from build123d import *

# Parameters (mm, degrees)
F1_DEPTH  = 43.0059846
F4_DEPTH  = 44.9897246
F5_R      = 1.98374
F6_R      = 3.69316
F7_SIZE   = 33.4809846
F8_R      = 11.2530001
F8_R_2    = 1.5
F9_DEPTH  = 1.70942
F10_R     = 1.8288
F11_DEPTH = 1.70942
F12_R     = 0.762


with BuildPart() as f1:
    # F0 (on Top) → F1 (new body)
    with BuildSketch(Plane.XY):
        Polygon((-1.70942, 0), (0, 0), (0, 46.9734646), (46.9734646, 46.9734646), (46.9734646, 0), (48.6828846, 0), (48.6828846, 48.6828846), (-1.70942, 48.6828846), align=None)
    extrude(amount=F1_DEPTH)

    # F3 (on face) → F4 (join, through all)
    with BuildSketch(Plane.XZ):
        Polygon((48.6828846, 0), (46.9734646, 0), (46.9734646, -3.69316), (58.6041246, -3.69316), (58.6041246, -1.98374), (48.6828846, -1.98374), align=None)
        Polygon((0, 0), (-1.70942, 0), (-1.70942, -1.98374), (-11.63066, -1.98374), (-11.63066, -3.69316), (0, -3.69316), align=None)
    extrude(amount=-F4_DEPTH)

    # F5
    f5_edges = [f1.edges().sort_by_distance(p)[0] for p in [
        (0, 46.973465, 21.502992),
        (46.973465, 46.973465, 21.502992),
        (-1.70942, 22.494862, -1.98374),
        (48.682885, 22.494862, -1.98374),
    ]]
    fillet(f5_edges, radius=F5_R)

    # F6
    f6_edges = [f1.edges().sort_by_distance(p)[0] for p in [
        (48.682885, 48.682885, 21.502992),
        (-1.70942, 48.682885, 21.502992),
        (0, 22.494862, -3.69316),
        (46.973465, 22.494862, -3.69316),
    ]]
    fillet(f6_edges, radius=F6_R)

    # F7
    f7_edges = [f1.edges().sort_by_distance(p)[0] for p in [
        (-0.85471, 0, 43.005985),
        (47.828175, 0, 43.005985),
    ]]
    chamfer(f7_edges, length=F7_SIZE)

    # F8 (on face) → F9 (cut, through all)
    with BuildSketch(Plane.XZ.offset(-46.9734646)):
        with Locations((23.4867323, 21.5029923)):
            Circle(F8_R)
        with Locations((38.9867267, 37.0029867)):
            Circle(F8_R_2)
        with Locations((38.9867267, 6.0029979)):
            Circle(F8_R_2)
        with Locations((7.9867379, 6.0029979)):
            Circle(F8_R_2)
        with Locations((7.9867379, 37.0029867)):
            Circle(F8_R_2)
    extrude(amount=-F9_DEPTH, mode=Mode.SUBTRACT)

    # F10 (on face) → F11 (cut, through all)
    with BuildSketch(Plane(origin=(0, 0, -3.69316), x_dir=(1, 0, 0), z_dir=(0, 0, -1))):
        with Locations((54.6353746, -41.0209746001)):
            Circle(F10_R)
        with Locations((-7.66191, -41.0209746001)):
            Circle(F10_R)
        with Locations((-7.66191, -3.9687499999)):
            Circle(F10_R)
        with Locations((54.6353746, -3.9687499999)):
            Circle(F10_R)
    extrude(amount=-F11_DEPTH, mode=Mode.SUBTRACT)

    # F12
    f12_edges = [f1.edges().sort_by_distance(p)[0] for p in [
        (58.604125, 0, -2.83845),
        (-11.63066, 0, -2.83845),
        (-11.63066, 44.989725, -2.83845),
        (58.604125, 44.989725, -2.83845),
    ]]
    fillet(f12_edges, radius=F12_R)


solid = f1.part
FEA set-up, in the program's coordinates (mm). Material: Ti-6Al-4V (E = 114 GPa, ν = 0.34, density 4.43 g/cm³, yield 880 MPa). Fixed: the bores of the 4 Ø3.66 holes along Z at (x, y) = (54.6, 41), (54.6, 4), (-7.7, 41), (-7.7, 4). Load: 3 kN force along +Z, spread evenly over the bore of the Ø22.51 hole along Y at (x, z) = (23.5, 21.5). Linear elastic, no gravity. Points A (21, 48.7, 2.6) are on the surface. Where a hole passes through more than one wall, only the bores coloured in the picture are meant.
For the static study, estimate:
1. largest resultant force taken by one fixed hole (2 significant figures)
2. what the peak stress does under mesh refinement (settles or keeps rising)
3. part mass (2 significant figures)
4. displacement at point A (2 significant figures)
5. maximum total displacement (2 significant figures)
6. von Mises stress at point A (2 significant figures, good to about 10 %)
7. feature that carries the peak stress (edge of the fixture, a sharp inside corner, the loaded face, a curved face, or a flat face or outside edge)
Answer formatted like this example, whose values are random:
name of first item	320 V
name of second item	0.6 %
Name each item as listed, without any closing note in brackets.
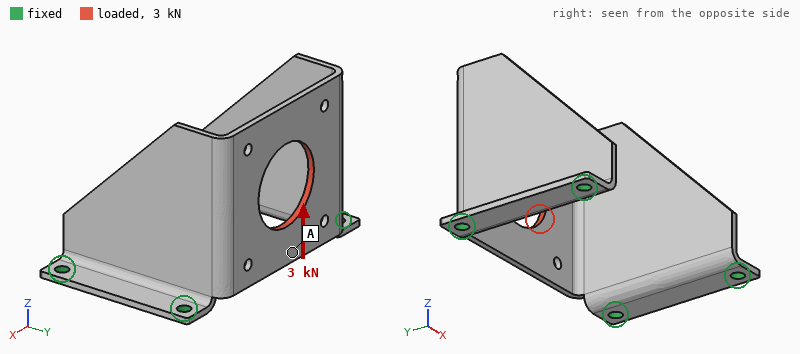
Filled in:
largest resultant force taken by one fixed hole	1.9 kN
what the peak stress does under mesh refinement	keeps rising
part mass	43 g
displacement at point A	0.22 mm
maximum total displacement	0.29 mm
von Mises stress at point A	88 MPa
feature that carries the peak stress	edge of the fixture
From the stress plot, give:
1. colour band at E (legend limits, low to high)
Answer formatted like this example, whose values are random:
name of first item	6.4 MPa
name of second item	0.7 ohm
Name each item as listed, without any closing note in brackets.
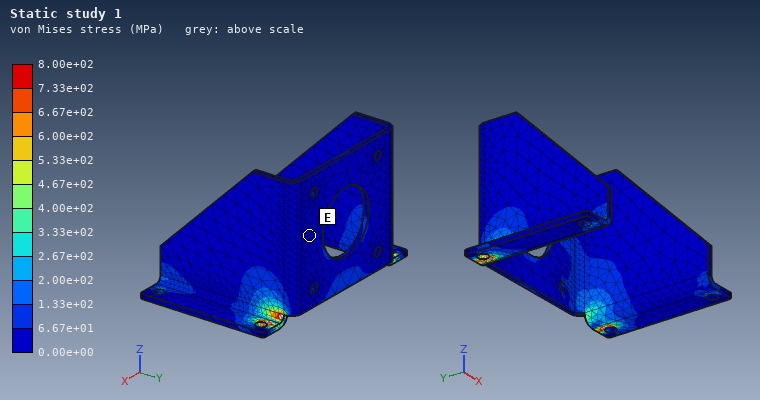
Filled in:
colour band at E	0.00e+00 to 6.67e+01 MPa
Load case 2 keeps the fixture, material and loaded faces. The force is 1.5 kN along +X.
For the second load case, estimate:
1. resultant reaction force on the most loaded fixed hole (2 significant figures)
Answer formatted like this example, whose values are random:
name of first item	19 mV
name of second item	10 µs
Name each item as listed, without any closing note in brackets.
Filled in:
resultant reaction force on the most loaded fixed hole	1.1 kN
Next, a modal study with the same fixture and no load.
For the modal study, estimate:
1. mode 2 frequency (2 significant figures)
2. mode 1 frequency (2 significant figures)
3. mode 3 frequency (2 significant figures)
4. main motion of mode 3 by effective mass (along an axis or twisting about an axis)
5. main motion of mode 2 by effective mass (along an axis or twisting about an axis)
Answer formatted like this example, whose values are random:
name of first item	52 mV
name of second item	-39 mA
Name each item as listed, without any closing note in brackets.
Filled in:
mode 2 frequency	2000 Hz
mode 1 frequency	1700 Hz
mode 3 frequency	2800 Hz
main motion of mode 3 by effective mass	along Y
main motion of mode 2 by effective mass	along X
